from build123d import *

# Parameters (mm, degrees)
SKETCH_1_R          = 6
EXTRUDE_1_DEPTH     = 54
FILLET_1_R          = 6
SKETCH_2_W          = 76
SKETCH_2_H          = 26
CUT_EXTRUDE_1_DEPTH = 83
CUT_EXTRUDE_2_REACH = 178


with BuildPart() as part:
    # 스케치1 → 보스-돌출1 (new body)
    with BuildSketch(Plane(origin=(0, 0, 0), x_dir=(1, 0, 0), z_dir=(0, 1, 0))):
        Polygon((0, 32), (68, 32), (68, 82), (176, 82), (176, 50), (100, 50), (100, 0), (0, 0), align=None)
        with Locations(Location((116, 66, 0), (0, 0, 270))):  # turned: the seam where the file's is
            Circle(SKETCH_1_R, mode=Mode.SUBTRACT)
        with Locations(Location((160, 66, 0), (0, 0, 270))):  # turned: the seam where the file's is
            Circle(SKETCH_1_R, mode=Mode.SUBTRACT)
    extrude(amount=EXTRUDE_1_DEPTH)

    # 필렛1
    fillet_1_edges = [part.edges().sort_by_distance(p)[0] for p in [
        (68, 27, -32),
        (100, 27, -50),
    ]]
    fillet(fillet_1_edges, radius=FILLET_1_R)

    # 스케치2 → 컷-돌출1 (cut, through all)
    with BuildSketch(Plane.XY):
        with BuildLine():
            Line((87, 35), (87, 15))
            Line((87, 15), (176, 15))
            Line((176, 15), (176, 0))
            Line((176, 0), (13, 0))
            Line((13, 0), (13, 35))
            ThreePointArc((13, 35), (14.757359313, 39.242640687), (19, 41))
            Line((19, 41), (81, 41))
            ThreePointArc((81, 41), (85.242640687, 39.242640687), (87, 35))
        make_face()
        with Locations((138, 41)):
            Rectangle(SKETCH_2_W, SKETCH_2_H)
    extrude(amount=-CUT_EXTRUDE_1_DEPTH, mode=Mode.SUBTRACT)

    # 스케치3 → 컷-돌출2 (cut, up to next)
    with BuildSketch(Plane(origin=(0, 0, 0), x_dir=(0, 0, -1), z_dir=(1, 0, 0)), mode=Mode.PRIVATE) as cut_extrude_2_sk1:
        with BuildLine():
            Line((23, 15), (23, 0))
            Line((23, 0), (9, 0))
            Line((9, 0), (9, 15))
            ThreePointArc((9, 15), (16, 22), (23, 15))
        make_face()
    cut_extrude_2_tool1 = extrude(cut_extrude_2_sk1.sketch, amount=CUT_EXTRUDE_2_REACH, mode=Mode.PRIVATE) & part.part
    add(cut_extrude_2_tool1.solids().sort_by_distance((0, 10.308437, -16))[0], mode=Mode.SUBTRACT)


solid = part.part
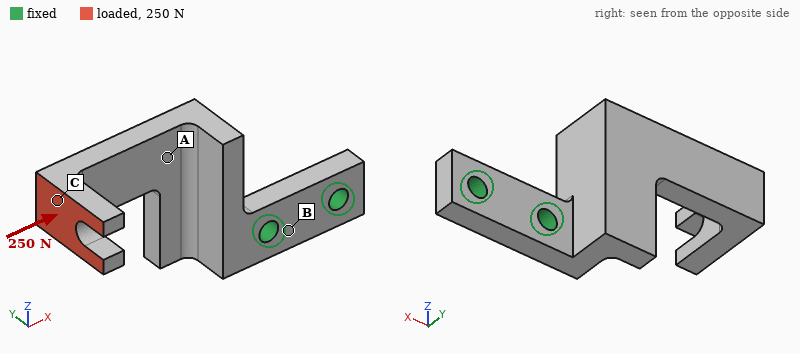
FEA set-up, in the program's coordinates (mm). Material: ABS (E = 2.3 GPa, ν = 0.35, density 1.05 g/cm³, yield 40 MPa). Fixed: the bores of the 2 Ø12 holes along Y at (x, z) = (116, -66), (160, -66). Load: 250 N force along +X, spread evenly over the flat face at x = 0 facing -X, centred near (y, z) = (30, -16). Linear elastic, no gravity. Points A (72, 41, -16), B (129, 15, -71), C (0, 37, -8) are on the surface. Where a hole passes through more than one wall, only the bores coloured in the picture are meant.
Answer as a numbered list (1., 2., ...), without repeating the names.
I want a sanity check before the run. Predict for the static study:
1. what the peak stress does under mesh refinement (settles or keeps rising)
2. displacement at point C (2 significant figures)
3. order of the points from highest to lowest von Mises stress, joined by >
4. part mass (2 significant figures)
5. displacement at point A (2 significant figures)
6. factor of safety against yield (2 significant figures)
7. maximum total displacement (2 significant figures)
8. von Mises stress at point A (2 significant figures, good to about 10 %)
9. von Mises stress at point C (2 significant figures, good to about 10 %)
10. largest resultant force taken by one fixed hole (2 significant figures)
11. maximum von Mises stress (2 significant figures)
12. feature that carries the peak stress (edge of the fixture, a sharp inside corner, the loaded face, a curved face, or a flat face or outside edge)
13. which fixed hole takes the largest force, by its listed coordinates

1. settles
2. 1.5 mm
3. A > C > B
4. 140 g
5. 0.65 mm
6. 1.9
7. 2.2 mm
8. 4.7 MPa
9. 2.4 MPa
10. 260 N
11. 21 MPa
12. a curved face
13. (116, -66)
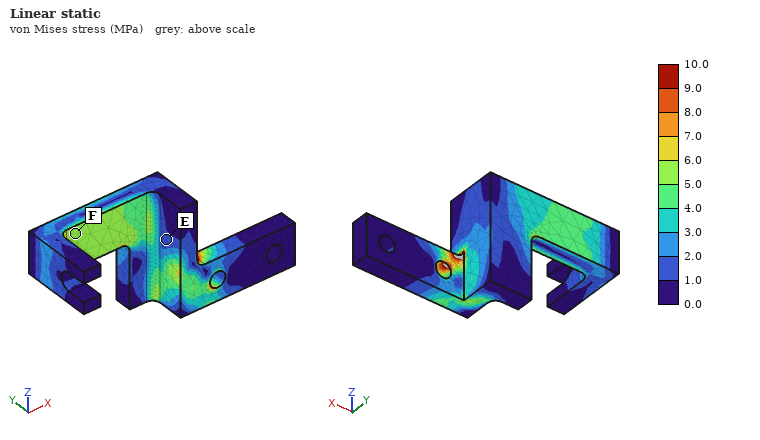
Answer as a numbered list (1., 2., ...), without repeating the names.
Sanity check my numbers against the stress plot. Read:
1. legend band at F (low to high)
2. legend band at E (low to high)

1. 5.0 to 6.0 MPa
2. 1.0 to 2.0 MPa
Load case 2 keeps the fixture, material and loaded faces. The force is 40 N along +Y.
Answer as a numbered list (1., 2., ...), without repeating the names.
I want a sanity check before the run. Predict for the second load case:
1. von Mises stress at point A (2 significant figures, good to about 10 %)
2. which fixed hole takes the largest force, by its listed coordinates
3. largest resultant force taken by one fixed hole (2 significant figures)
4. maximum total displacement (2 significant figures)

1. 2.7 MPa
2. (116, -66)
3. 50 N
4. 2.0 mm
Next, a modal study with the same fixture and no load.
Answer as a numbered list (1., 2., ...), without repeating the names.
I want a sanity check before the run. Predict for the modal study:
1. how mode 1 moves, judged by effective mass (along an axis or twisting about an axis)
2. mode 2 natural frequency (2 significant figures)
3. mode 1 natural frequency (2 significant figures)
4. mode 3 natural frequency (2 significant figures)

1. along Y
2. 230 Hz
3. 140 Hz
4. 440 Hz
